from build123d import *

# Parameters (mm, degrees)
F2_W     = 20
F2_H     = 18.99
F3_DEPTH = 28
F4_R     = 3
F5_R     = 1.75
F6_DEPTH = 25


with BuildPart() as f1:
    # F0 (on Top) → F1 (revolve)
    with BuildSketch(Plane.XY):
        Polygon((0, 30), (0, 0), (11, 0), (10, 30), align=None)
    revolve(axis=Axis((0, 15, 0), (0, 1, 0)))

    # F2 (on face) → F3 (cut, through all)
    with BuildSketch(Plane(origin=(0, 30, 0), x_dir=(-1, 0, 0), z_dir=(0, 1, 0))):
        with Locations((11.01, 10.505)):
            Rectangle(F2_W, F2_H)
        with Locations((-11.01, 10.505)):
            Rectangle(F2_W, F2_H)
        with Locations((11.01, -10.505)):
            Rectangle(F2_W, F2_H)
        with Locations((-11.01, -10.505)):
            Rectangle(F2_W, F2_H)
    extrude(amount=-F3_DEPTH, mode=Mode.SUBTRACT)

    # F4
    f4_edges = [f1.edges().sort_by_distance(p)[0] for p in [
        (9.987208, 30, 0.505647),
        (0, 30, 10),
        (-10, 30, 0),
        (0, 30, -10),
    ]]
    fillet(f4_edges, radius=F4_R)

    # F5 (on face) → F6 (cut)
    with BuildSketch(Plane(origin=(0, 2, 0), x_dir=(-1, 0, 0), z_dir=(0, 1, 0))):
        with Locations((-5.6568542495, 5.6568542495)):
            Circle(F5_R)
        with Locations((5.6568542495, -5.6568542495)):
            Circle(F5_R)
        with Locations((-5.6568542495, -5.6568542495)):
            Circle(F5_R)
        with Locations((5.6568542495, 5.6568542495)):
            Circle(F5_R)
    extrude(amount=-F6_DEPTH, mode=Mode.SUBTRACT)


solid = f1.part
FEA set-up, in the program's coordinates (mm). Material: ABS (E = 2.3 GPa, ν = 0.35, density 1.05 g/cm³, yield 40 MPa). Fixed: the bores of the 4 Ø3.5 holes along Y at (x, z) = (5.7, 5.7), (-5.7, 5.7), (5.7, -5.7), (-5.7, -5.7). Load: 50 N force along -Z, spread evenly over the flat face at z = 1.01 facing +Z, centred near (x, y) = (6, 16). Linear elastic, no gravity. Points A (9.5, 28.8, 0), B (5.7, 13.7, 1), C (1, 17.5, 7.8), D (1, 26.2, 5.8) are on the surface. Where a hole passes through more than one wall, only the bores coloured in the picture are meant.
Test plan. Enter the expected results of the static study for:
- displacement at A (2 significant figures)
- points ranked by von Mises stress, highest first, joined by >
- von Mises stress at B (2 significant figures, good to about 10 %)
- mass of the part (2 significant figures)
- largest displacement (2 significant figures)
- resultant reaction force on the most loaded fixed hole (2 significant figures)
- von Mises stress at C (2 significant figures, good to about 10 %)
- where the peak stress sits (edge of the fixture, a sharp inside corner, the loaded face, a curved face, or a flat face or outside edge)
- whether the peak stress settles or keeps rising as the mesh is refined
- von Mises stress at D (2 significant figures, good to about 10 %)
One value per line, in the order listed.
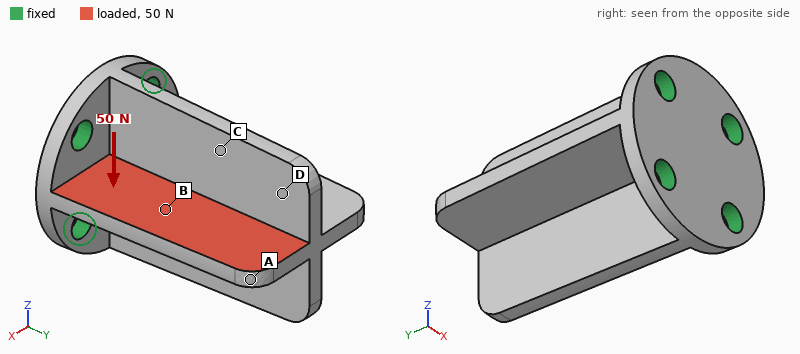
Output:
0.49 mm
B > C > D > A
5.8 MPa
3.1 g
0.50 mm
37 N
4.1 MPa
edge of the fixture
keeps rising
2.3 MPa
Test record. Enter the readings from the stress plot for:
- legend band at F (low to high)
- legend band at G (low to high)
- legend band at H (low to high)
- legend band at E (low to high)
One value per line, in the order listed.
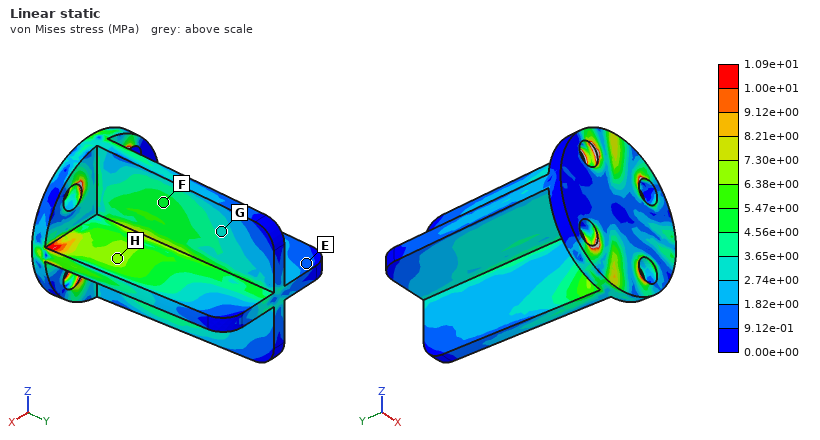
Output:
4.56e+00 to 5.47e+00 MPa
2.74e+00 to 3.65e+00 MPa
6.38e+00 to 7.30e+00 MPa
9.12e-01 to 1.82e+00 MPa
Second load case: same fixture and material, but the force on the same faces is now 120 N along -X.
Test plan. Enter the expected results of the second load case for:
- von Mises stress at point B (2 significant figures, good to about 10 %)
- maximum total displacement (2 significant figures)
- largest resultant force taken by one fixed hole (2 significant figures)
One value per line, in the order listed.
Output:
6.8 MPa
0.47 mm
77 N
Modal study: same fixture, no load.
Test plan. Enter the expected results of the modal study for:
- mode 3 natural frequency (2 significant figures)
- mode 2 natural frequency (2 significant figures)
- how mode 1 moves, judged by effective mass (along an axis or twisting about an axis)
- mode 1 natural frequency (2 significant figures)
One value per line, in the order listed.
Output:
2200 Hz
2200 Hz
twisting about Y
1900 Hz
